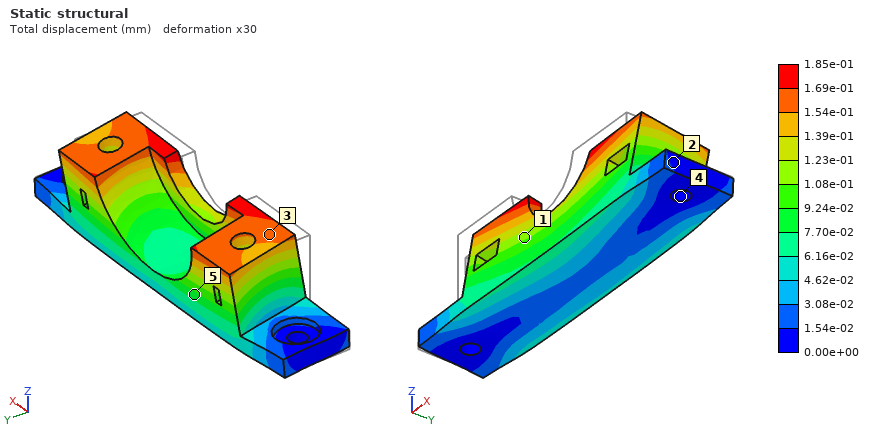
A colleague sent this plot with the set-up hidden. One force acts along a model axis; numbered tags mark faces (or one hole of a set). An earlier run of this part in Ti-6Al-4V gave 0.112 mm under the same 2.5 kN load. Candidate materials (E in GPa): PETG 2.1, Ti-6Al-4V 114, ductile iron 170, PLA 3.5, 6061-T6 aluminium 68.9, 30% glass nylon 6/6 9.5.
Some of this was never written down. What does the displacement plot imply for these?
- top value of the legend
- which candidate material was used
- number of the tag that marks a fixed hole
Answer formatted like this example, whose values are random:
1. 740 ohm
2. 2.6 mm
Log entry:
1. 1.85e-01 mm
2. 6061-T6 aluminium
3. 4
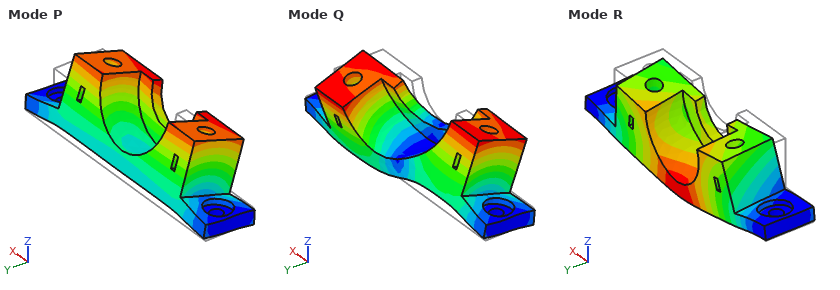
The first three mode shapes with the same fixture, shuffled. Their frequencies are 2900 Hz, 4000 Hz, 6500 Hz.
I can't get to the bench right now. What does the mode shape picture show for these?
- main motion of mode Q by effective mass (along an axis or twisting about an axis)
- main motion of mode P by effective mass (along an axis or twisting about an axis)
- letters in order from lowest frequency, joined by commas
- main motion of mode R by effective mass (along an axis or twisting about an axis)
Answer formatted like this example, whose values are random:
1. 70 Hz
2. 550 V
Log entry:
1. twisting about Z
2. along Y
3. P, R, Q
4. along Z
